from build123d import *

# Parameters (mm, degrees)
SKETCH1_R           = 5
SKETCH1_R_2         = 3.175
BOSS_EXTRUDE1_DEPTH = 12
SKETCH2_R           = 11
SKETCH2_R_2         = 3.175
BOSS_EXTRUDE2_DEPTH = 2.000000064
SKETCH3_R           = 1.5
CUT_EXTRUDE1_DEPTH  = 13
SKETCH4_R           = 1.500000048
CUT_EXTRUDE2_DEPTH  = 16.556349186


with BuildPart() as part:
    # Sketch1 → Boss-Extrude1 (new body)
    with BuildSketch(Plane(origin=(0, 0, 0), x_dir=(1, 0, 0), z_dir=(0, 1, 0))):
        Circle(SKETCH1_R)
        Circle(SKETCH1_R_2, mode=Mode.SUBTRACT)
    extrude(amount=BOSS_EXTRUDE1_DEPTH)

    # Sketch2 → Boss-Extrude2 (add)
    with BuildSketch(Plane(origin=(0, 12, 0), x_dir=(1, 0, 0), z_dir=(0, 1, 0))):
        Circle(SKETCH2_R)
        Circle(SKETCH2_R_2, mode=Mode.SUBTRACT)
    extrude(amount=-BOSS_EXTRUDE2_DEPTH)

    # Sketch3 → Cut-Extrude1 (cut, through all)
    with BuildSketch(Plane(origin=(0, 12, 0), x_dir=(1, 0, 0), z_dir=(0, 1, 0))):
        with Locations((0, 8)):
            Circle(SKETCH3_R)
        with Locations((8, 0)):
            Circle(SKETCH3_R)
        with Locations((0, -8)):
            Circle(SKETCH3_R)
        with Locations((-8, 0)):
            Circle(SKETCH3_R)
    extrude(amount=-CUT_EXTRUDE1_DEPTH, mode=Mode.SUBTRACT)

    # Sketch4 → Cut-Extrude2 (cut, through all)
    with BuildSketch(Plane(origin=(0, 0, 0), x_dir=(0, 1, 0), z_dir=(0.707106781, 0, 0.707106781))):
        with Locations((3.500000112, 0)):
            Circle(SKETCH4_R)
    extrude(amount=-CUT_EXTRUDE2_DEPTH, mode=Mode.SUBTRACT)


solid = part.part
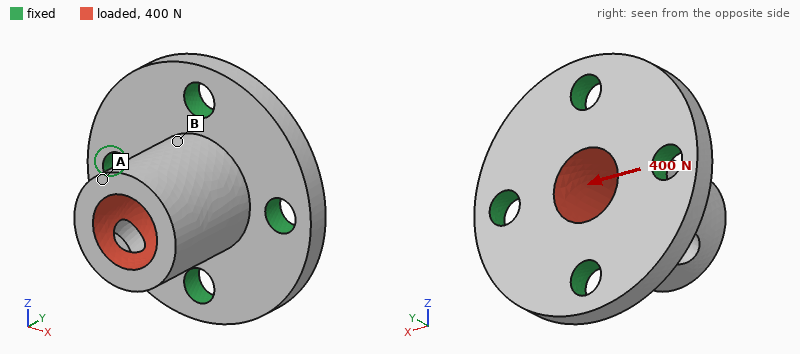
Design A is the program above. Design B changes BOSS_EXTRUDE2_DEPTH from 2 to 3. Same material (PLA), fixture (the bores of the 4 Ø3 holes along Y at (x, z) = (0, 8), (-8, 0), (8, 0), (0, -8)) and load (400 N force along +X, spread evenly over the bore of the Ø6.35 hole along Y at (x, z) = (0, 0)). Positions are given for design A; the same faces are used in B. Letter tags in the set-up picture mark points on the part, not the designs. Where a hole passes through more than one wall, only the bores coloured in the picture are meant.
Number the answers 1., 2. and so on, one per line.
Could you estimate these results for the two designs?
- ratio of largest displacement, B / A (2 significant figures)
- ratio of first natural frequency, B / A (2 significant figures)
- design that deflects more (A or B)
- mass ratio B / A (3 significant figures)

1. 0.61
2. 1.3
3. A
4. 1.25
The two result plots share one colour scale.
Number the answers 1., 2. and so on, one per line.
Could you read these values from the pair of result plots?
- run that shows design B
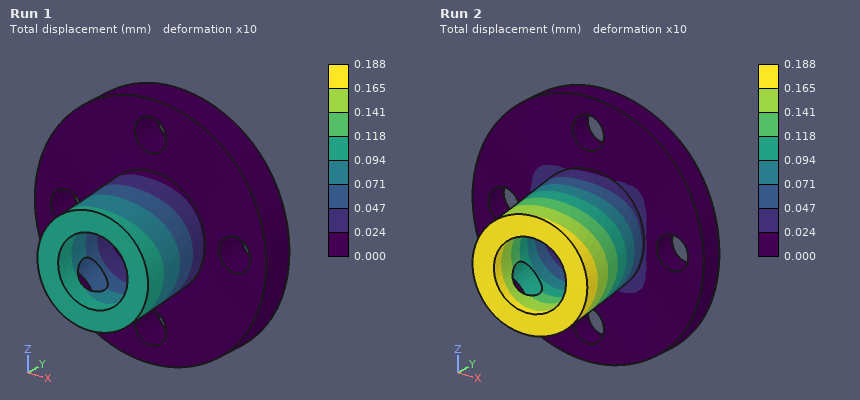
1. Run 1
